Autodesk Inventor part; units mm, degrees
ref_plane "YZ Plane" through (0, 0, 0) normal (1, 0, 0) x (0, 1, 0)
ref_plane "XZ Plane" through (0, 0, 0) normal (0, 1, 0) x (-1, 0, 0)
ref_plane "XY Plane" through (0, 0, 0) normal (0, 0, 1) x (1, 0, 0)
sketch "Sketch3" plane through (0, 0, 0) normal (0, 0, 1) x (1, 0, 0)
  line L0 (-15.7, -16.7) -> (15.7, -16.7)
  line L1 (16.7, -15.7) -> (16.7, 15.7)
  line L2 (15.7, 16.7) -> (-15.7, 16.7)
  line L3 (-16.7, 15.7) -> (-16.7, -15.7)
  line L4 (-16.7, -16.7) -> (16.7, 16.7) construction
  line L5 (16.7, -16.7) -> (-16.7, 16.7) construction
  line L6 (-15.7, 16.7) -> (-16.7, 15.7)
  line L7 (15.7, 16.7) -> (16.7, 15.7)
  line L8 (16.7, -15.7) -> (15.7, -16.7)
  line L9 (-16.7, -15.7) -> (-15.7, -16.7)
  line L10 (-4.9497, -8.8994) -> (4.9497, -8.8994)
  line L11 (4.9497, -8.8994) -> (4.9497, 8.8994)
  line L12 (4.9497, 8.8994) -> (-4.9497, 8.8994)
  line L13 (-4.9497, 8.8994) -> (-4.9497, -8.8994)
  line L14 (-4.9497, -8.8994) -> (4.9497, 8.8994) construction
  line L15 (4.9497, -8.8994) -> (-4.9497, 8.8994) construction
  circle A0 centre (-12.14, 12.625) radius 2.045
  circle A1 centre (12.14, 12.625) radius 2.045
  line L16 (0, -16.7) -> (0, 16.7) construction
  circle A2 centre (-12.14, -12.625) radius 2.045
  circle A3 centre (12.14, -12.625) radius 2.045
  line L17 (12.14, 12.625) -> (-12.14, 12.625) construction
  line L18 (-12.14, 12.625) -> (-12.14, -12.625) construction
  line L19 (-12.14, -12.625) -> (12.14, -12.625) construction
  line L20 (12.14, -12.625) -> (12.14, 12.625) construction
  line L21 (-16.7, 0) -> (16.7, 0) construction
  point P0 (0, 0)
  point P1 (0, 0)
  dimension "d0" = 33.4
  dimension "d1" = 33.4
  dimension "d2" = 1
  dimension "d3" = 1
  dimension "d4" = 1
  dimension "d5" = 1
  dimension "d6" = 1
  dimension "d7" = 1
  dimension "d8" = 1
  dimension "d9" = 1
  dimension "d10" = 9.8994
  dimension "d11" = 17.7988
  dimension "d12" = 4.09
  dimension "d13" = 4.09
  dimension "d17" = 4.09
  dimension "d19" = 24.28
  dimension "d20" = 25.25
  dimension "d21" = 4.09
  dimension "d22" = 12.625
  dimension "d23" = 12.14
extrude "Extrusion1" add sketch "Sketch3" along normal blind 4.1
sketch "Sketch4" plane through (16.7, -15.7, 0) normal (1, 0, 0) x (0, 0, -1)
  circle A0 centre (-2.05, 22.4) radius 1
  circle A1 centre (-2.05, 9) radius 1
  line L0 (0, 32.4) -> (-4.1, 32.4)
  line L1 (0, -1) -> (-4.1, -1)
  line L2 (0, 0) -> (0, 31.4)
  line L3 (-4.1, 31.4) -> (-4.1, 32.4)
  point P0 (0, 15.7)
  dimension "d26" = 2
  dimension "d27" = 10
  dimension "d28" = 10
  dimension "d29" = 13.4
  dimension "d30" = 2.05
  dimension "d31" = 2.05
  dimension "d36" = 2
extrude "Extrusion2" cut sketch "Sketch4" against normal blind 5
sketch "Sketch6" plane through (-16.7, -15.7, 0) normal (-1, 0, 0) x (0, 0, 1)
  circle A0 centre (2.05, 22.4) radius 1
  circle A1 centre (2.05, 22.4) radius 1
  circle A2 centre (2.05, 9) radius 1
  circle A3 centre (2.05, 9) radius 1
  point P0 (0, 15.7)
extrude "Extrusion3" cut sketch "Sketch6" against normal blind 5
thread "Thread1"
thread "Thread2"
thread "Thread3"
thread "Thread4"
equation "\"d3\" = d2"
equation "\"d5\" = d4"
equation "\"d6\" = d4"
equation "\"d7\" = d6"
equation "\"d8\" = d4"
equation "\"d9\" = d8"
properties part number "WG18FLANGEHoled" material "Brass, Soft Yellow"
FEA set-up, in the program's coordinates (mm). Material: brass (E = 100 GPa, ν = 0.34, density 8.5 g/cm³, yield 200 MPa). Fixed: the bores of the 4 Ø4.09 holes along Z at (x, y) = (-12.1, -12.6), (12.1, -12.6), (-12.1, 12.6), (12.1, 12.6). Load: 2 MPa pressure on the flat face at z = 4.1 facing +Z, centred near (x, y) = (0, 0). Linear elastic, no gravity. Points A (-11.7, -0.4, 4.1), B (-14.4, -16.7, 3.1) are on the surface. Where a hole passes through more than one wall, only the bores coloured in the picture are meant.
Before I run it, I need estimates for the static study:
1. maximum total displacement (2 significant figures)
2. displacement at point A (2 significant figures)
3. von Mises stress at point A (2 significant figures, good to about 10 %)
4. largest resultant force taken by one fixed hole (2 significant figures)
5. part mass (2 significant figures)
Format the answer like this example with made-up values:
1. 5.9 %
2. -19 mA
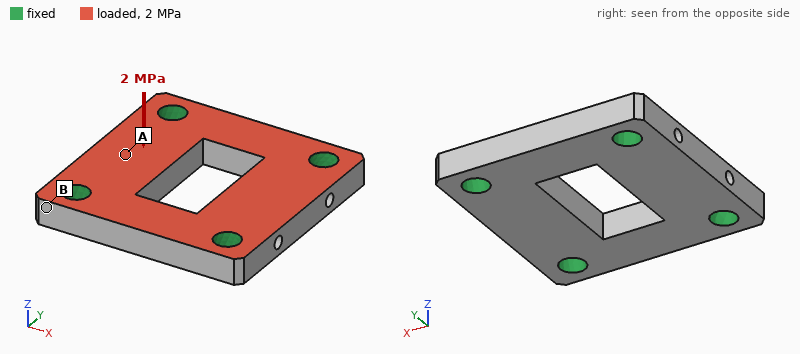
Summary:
1. 5.9 µm
2. 4.1 µm
3. 15 MPa
4. 440 N
5. 30 g
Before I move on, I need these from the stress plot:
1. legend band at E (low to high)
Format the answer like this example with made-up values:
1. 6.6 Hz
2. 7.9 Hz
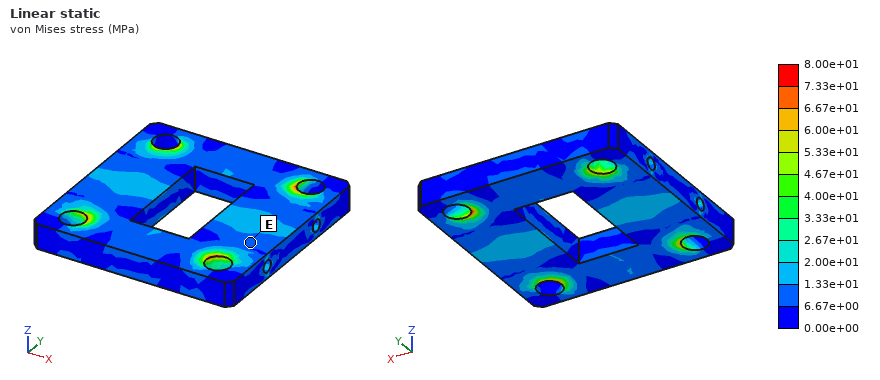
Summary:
1. 6.67e+00 to 1.33e+01 MPa
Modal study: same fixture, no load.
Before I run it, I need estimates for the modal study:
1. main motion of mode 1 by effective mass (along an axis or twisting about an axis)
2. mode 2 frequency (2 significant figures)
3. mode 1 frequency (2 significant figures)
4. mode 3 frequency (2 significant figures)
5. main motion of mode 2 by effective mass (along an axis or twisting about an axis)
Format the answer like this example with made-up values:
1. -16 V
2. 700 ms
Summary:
1. along Z
2. 22 kHz
3. 20 kHz
4. 25 kHz
5. twisting about Y
